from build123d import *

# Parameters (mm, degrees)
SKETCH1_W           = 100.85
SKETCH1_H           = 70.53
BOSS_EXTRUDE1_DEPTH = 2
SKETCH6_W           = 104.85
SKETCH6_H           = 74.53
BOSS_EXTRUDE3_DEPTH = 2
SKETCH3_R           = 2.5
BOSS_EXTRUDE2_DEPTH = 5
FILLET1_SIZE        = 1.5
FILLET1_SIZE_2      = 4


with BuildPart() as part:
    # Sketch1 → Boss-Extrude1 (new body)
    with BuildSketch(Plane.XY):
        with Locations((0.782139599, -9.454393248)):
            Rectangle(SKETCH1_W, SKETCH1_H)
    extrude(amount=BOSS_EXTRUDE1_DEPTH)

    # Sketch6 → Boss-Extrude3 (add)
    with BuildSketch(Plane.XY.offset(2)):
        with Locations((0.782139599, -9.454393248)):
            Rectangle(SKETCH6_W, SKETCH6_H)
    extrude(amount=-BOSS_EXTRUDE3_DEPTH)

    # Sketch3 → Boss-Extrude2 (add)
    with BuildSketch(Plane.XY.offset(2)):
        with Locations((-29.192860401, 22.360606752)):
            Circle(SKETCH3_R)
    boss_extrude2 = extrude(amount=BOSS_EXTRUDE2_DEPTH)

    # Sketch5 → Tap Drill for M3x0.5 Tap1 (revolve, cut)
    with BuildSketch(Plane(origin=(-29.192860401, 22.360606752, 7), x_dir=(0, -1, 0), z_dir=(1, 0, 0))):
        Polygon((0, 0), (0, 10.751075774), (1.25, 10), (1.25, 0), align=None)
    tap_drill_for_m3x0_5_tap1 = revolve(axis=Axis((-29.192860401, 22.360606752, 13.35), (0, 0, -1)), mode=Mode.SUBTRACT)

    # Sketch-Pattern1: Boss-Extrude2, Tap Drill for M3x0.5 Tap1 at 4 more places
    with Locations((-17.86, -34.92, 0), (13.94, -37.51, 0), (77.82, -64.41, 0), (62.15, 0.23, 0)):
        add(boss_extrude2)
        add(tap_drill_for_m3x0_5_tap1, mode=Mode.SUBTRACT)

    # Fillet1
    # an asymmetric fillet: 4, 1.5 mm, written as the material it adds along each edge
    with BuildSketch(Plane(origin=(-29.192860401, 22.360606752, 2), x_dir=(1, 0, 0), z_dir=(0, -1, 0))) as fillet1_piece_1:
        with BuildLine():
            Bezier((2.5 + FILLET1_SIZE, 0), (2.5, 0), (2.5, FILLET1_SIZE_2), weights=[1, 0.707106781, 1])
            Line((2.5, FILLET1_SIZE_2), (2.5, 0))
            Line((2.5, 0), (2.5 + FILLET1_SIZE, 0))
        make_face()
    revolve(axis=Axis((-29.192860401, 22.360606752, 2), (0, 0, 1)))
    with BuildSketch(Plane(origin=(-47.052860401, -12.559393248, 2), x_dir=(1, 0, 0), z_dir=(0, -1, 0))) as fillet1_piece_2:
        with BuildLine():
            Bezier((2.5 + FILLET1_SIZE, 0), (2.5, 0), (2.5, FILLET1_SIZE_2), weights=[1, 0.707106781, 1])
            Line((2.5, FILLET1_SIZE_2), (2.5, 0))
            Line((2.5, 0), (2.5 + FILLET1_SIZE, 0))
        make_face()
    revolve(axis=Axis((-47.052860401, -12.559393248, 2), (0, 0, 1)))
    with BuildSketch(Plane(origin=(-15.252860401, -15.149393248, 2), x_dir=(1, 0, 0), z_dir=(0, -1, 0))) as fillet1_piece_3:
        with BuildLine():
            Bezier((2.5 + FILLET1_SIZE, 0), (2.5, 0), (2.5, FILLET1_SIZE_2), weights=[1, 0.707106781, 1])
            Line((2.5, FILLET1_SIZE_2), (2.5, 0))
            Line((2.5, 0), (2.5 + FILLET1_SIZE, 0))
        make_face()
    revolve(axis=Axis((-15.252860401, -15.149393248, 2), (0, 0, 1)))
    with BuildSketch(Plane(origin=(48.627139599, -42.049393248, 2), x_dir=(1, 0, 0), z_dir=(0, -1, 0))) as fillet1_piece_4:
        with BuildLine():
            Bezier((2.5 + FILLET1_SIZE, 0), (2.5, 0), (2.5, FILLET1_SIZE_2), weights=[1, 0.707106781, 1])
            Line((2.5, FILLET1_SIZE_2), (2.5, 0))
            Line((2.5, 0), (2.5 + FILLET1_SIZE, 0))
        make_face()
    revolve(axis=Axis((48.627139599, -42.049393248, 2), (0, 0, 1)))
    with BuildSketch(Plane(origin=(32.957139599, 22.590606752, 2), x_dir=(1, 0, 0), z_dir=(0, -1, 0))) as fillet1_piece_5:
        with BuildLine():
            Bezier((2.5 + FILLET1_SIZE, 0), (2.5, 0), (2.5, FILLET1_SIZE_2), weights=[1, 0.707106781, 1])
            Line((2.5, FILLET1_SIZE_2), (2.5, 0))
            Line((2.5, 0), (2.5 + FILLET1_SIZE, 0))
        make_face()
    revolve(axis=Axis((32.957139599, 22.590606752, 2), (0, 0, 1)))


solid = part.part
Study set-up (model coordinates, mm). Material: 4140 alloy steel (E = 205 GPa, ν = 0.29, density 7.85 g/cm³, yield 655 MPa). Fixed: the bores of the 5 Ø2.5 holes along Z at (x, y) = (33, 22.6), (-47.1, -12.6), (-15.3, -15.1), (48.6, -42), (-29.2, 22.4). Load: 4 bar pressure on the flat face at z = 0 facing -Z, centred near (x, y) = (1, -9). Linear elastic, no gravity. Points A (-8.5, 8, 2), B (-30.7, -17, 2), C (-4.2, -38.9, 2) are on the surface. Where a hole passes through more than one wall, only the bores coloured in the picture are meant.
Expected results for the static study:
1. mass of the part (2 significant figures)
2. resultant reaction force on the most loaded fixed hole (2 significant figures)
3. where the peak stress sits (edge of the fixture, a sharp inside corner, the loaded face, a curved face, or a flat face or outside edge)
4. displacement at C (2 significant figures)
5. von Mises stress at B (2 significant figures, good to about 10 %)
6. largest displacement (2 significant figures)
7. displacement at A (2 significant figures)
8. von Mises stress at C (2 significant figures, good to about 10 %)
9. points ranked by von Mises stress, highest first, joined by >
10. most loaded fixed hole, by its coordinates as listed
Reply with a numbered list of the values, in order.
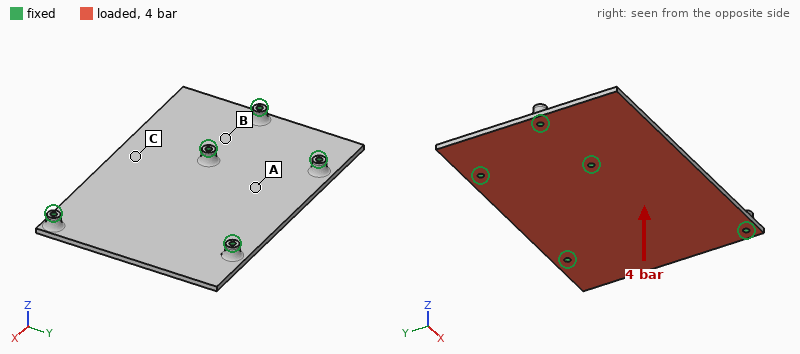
1. 130 g
2. 1.1 kN
3. a curved face
4. 0.25 mm
5. 130 MPa
6. 0.36 mm
7. 0.059 mm
8. 79 MPa
9. B > C > A
10. (-15.3, -15.1)
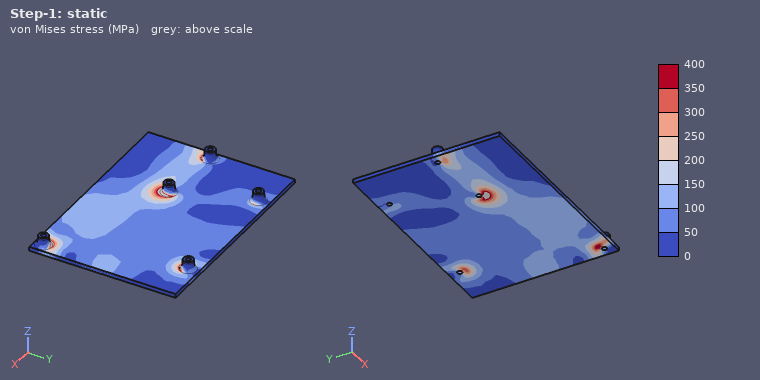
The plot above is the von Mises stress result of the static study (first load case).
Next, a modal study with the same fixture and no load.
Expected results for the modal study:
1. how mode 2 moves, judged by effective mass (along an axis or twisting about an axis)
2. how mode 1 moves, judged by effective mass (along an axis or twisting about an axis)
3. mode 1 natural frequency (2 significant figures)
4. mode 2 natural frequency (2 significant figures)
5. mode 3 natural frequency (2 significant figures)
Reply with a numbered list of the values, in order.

1. along Z
2. along Z
3. 1700 Hz
4. 2100 Hz
5. 2500 Hz
